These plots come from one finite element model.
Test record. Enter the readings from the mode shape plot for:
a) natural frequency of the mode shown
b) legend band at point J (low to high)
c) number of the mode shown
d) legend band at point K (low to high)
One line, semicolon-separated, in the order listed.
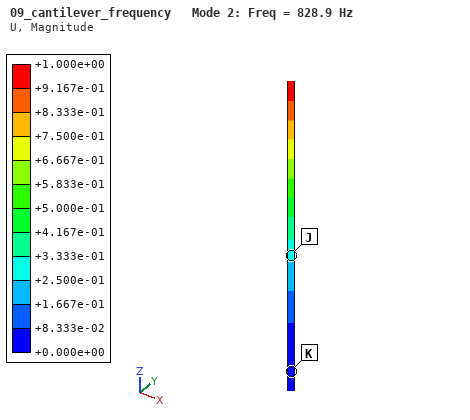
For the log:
828.9 Hz; +2.500e-01 to +3.333e-01; 2; +0.000e+00 to +8.333e-02
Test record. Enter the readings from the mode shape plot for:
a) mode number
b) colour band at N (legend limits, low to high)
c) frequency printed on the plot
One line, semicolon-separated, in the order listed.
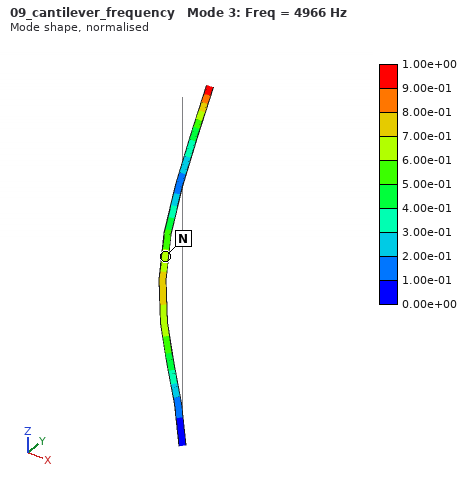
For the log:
3; 6.00e-01 to 7.00e-01; 4966 Hz
